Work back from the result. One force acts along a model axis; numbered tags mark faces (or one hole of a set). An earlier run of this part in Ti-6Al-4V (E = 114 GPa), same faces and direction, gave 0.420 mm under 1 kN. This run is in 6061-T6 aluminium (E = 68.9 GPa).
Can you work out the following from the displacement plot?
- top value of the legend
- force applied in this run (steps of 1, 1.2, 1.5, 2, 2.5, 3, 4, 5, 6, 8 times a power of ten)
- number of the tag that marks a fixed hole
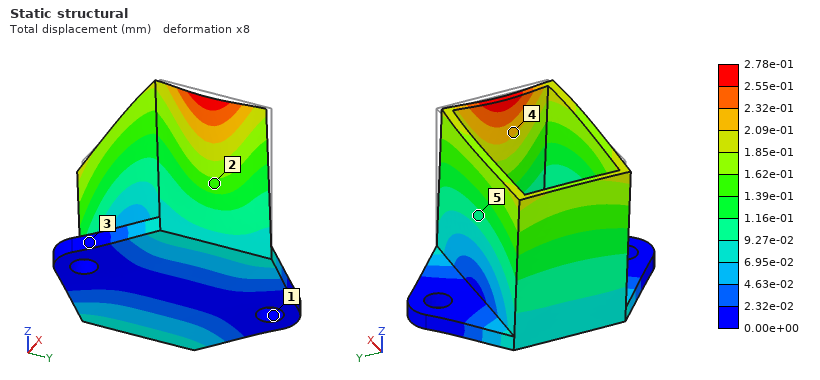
2.78e-01 mm
400 N
1
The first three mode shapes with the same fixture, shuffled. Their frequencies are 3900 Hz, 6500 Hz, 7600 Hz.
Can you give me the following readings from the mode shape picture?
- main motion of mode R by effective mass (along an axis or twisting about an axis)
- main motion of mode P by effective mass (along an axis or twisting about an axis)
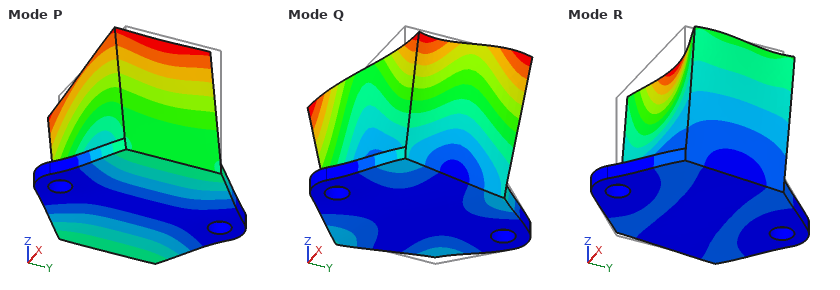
along Y
along X
